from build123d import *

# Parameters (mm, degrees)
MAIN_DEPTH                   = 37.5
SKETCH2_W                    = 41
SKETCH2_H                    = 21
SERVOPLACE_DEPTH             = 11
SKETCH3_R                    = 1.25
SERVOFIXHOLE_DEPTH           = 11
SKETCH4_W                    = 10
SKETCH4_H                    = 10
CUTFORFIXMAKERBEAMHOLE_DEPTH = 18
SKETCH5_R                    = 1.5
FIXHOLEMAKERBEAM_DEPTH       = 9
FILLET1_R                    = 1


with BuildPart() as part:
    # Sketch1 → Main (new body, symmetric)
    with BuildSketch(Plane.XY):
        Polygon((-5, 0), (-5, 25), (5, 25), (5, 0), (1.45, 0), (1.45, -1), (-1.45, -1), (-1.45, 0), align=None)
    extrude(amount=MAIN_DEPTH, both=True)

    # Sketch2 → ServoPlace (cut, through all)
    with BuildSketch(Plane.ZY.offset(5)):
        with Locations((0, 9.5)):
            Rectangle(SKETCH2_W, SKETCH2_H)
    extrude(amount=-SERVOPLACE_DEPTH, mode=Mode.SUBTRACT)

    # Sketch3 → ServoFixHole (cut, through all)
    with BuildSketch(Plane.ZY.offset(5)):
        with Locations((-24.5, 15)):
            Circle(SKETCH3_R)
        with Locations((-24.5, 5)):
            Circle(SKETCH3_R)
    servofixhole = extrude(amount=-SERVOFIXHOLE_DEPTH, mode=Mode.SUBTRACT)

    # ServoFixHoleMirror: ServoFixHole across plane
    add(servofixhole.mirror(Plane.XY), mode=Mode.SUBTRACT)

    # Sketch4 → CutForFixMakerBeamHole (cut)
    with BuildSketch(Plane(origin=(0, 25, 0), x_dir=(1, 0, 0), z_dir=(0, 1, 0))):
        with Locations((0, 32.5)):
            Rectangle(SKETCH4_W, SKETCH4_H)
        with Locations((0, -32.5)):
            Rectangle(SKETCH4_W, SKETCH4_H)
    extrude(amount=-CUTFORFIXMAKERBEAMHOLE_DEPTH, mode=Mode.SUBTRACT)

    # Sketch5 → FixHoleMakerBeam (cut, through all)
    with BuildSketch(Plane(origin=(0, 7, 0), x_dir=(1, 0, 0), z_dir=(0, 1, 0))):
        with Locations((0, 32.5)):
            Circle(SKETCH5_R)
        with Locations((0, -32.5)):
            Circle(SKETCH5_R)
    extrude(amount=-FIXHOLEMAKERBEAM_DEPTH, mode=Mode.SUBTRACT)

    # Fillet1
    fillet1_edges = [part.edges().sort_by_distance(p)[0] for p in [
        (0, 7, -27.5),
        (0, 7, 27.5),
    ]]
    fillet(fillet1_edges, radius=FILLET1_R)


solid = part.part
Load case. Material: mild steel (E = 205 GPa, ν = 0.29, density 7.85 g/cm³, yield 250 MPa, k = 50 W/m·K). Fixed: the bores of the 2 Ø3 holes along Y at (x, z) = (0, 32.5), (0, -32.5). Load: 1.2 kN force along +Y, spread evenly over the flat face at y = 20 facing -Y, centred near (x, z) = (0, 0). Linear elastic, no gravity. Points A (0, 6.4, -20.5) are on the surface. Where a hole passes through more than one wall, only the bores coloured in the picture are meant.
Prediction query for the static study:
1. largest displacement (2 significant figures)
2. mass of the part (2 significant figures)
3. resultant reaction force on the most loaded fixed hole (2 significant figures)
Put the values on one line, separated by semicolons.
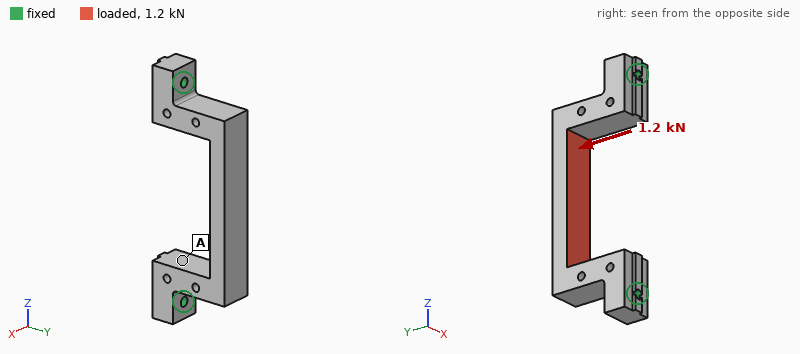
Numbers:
23 µm; 53 g; 740 N
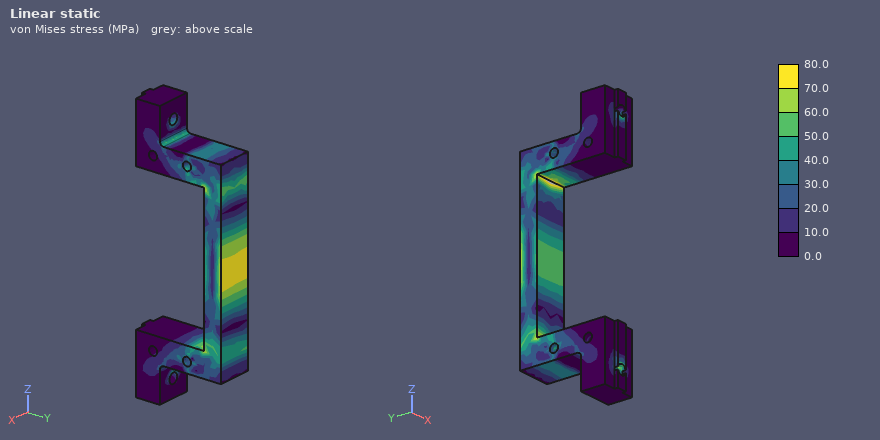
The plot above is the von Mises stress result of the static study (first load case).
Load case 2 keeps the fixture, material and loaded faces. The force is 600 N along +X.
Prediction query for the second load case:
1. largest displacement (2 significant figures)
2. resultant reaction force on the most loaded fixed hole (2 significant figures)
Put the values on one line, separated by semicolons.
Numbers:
29 µm; 300 N
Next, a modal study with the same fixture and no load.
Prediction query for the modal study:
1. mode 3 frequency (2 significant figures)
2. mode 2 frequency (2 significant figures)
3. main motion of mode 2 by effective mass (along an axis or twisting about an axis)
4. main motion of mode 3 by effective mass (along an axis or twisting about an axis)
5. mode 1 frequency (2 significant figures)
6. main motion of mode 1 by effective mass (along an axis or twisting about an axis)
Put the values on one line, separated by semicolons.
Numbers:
8800 Hz; 6800 Hz; along Z; twisting about Y; 4900 Hz; along X
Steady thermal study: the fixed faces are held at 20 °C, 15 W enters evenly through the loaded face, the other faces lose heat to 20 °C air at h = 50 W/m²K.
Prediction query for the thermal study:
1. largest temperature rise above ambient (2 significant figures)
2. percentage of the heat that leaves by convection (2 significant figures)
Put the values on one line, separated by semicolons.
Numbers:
70 K; 32 %
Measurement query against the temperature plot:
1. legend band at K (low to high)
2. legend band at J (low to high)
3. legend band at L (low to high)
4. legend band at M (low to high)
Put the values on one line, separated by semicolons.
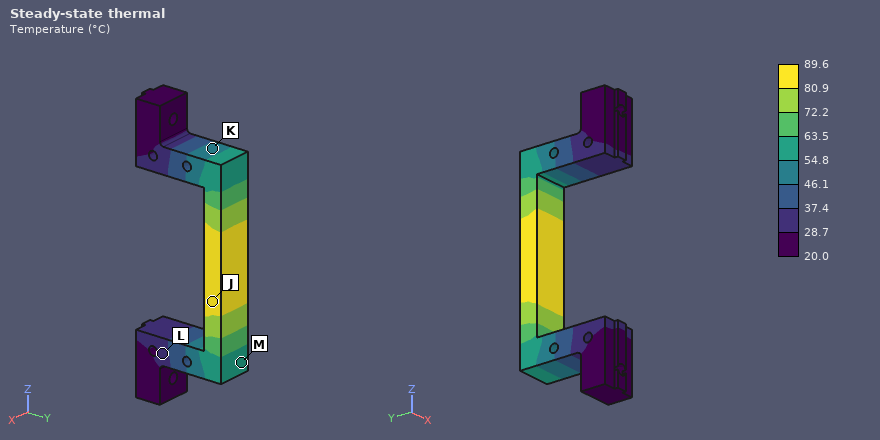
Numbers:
46.1 to 54.8 °C; 80.9 to 89.6 °C; 28.7 to 37.4 °C; 54.8 to 63.5 °C
